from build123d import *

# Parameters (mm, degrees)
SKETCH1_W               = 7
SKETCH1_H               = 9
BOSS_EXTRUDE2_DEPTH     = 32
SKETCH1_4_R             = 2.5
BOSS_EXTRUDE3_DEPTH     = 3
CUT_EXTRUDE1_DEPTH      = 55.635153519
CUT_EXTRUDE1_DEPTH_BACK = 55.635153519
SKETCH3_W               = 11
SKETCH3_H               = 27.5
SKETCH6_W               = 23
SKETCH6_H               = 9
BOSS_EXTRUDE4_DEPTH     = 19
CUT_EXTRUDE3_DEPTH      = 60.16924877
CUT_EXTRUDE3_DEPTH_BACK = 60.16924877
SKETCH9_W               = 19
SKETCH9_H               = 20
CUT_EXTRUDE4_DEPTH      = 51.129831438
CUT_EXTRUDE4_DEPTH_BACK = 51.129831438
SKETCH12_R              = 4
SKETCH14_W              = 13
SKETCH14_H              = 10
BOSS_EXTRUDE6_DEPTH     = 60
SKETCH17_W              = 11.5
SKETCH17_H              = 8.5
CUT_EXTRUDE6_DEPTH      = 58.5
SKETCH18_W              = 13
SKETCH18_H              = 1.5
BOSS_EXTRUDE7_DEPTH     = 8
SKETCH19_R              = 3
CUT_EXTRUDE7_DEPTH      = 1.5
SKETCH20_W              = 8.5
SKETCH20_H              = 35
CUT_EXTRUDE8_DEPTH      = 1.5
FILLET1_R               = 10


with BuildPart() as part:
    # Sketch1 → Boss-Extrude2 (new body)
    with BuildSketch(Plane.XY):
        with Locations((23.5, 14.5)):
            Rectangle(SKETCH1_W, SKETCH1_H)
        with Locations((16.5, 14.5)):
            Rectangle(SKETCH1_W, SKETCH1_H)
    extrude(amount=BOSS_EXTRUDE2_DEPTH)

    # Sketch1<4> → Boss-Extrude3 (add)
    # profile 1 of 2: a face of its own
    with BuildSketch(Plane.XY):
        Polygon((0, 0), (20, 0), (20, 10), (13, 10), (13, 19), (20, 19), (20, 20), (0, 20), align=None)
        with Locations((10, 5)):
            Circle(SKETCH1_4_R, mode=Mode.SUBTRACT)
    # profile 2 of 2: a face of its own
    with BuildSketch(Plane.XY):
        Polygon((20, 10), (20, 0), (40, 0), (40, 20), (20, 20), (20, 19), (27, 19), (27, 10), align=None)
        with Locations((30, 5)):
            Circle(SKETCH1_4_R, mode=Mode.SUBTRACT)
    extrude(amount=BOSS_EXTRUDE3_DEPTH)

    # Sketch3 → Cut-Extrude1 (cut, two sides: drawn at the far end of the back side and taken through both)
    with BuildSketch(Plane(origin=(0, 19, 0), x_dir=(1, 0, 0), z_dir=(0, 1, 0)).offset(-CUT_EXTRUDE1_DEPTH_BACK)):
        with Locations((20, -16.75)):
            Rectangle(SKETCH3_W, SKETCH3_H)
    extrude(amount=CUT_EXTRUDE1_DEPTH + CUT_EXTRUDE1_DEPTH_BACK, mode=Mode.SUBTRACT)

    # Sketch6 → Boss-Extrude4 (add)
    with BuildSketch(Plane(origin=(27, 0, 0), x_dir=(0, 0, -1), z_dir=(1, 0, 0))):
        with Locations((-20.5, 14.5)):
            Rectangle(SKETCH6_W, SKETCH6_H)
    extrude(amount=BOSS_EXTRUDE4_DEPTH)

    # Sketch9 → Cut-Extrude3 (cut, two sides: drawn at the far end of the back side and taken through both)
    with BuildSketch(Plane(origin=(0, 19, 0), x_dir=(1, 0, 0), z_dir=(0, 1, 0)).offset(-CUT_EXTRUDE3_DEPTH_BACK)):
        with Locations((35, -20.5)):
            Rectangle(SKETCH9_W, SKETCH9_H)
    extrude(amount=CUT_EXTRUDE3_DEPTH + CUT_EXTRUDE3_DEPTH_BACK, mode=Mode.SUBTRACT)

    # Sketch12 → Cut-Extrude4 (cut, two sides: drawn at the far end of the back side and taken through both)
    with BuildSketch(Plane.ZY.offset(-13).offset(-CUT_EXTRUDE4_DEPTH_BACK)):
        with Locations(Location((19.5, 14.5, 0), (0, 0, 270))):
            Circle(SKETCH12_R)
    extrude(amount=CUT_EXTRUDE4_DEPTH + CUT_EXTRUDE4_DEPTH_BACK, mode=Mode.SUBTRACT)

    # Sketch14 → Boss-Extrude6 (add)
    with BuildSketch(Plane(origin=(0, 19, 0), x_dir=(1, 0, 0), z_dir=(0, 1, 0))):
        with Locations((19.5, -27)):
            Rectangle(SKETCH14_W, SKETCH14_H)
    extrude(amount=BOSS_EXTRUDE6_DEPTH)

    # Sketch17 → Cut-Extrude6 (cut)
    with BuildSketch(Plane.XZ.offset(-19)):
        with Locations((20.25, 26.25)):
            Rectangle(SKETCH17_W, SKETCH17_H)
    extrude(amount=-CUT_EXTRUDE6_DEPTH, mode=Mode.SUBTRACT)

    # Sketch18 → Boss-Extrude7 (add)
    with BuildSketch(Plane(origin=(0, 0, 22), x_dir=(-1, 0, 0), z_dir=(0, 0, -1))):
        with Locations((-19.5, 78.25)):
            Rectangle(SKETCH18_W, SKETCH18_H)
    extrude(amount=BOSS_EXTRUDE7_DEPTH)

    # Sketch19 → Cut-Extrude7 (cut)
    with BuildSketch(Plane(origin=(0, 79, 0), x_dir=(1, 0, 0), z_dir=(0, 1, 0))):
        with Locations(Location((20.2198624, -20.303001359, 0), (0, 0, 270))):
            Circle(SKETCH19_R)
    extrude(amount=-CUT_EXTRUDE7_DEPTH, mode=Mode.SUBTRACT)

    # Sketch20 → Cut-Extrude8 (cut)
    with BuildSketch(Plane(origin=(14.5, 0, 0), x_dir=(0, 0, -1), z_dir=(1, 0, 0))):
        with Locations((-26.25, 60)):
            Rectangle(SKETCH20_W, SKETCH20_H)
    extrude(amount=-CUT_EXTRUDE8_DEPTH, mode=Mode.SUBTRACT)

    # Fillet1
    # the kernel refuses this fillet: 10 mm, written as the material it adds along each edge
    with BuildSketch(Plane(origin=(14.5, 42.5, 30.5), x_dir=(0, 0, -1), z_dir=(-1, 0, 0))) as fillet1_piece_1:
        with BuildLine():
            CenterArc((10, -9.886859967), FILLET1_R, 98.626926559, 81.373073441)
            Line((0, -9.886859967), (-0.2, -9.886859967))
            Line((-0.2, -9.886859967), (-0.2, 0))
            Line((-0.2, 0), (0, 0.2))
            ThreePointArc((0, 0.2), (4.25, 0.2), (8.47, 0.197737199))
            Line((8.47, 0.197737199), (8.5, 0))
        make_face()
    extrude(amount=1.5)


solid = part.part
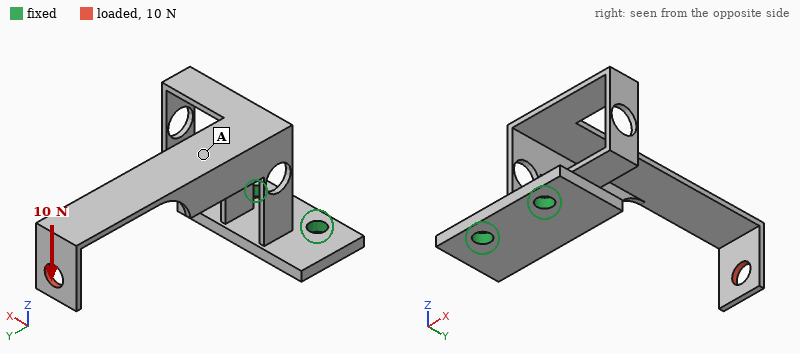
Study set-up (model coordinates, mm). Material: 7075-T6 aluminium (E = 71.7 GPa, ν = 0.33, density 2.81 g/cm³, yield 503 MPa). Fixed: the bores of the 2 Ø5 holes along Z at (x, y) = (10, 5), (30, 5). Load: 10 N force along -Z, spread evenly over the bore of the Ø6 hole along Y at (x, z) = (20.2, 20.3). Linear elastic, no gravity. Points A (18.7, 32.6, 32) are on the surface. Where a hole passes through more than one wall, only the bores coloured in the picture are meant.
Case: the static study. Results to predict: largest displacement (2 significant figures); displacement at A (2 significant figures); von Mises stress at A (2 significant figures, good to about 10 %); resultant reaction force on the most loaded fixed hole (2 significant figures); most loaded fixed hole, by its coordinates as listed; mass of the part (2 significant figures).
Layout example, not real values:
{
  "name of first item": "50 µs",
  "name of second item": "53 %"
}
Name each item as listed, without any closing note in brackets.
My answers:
{
  "largest displacement": "1.0 mm",
  "displacement at A": "0.16 mm",
  "von Mises stress at A": "12 MPa",
  "resultant reaction force on the most loaded fixed hole": "8.9 N",
  "most loaded fixed hole, by its coordinates as listed": "(30, 5)",
  "mass of the part": "15 g"
}
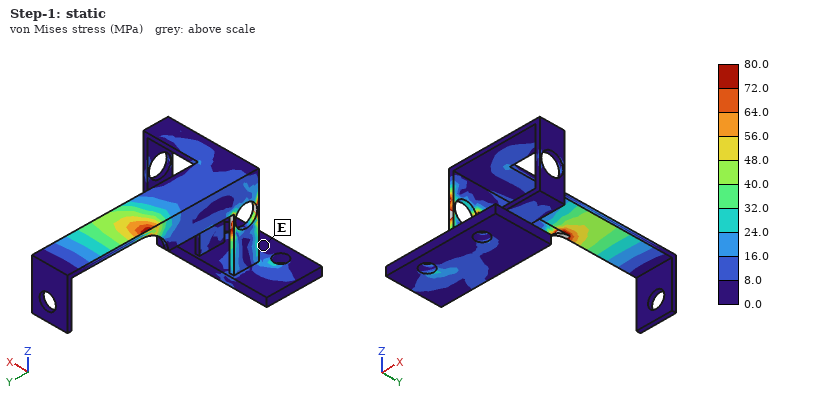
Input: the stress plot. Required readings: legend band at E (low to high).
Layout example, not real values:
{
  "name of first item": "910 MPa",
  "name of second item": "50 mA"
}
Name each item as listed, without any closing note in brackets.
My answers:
{
  "legend band at E": "0.0 to 8.0 MPa"
}
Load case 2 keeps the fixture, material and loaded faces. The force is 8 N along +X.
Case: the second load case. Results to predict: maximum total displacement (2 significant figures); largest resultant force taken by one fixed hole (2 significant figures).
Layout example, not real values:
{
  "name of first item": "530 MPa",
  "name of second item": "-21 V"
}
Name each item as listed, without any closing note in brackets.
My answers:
{
  "maximum total displacement": "0.97 mm",
  "largest resultant force taken by one fixed hole": "29 N"
}
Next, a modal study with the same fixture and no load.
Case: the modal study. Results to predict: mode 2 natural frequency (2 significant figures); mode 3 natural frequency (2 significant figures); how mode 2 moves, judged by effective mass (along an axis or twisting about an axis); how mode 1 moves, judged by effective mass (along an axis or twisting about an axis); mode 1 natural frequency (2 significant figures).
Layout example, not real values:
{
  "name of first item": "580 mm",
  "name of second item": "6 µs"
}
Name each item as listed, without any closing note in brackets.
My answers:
{
  "mode 2 natural frequency": "420 Hz",
  "mode 3 natural frequency": "680 Hz",
  "how mode 2 moves, judged by effective mass": "along Z",
  "how mode 1 moves, judged by effective mass": "along X",
  "mode 1 natural frequency": "320 Hz"
}
